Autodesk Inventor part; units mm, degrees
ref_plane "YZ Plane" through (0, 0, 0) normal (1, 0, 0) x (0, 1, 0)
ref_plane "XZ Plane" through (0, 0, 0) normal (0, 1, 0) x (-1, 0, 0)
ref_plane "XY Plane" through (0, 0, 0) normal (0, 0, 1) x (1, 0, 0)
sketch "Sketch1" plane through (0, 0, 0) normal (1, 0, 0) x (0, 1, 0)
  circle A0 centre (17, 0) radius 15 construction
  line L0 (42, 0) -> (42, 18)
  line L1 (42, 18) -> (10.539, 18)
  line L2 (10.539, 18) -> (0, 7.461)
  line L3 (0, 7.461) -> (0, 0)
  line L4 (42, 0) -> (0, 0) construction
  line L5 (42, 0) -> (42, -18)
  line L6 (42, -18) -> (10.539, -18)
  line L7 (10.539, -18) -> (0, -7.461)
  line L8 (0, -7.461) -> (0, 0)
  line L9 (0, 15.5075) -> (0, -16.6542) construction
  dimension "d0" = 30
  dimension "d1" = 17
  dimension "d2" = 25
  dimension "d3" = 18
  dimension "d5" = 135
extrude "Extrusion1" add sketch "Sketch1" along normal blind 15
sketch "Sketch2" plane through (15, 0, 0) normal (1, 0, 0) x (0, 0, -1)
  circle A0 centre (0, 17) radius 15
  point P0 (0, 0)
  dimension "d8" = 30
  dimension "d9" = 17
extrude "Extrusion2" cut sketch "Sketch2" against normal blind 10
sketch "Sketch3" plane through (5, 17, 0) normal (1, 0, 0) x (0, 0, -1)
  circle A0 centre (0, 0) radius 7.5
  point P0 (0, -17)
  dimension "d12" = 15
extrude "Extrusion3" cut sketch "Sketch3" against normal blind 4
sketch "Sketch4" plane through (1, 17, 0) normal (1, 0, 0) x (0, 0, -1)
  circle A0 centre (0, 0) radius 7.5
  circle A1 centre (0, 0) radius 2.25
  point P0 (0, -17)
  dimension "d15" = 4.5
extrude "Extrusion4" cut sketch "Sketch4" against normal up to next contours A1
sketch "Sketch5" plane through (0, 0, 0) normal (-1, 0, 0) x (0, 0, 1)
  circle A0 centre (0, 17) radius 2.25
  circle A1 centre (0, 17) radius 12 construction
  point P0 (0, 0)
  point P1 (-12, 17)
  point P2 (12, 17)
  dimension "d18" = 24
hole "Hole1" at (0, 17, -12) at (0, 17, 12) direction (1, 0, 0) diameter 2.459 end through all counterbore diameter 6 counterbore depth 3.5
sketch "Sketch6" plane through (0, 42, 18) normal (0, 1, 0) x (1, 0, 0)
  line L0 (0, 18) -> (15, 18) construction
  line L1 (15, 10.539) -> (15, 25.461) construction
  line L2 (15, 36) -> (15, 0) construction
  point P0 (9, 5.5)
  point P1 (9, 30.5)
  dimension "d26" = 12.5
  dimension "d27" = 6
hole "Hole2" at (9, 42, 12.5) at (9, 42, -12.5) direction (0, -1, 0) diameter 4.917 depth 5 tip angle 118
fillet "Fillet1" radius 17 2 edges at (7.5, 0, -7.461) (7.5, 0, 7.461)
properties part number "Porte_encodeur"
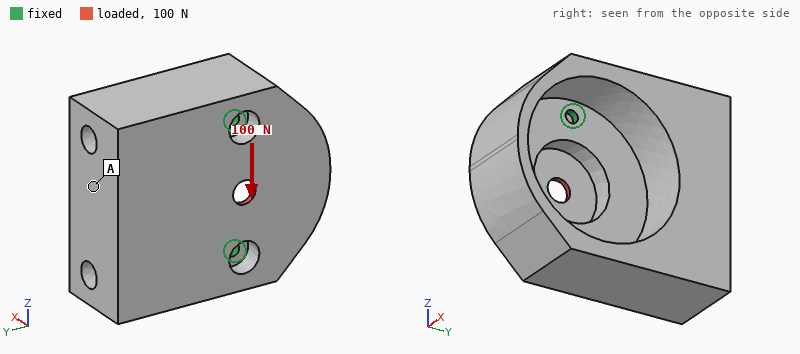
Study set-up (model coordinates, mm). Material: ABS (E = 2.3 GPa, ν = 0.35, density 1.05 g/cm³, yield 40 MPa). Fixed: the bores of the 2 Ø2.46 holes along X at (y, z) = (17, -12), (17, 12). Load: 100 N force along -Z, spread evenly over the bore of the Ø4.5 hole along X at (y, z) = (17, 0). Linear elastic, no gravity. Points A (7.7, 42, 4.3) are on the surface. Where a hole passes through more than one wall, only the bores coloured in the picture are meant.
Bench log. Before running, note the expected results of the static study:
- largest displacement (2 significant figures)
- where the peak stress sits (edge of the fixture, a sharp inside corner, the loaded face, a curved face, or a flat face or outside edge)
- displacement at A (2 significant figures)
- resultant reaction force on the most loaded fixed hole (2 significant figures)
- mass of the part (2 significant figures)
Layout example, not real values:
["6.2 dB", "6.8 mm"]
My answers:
["32 µm", "the loaded face", "5.5 µm", "52 N", "13 g"]
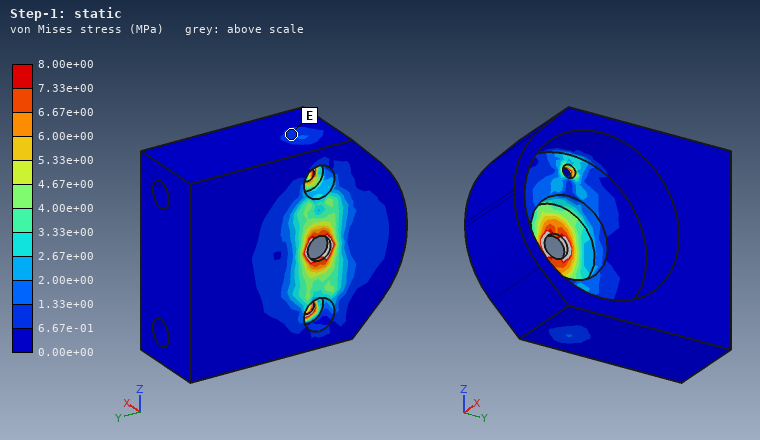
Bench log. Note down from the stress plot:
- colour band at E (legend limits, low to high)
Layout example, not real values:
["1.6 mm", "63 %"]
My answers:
["6.67e-01 to 1.33e+00 MPa"]
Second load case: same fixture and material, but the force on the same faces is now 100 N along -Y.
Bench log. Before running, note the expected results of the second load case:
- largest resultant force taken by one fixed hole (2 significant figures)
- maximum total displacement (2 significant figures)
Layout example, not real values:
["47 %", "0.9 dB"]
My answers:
["50 N", "0.44 mm"]
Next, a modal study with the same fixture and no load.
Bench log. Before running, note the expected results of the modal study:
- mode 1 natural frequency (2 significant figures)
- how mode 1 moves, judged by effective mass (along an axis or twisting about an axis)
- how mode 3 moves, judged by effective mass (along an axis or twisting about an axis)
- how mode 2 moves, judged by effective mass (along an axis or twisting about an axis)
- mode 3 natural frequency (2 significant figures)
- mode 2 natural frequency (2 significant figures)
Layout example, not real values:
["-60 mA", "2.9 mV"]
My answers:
["430 Hz", "along X", "along Z", "along Z", "3100 Hz", "2300 Hz"]
